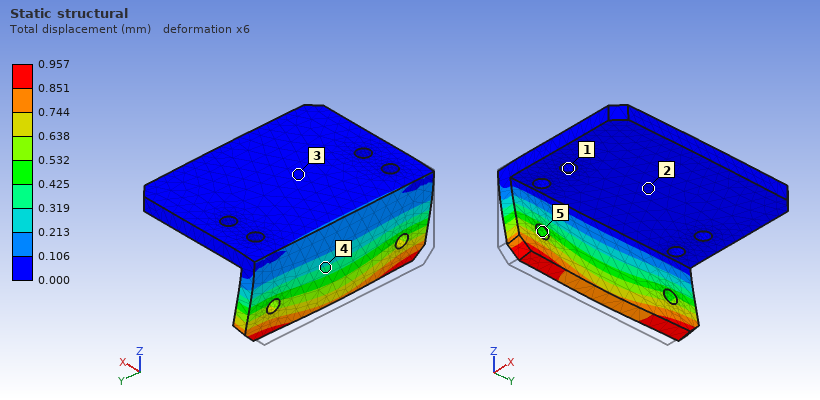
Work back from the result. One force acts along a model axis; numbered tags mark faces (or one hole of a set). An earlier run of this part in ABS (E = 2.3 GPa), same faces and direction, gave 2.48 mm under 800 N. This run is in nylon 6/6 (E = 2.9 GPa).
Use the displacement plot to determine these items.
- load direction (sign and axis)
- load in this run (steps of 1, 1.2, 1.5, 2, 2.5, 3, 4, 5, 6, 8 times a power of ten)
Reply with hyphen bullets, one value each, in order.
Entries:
- +X
- 400 N
